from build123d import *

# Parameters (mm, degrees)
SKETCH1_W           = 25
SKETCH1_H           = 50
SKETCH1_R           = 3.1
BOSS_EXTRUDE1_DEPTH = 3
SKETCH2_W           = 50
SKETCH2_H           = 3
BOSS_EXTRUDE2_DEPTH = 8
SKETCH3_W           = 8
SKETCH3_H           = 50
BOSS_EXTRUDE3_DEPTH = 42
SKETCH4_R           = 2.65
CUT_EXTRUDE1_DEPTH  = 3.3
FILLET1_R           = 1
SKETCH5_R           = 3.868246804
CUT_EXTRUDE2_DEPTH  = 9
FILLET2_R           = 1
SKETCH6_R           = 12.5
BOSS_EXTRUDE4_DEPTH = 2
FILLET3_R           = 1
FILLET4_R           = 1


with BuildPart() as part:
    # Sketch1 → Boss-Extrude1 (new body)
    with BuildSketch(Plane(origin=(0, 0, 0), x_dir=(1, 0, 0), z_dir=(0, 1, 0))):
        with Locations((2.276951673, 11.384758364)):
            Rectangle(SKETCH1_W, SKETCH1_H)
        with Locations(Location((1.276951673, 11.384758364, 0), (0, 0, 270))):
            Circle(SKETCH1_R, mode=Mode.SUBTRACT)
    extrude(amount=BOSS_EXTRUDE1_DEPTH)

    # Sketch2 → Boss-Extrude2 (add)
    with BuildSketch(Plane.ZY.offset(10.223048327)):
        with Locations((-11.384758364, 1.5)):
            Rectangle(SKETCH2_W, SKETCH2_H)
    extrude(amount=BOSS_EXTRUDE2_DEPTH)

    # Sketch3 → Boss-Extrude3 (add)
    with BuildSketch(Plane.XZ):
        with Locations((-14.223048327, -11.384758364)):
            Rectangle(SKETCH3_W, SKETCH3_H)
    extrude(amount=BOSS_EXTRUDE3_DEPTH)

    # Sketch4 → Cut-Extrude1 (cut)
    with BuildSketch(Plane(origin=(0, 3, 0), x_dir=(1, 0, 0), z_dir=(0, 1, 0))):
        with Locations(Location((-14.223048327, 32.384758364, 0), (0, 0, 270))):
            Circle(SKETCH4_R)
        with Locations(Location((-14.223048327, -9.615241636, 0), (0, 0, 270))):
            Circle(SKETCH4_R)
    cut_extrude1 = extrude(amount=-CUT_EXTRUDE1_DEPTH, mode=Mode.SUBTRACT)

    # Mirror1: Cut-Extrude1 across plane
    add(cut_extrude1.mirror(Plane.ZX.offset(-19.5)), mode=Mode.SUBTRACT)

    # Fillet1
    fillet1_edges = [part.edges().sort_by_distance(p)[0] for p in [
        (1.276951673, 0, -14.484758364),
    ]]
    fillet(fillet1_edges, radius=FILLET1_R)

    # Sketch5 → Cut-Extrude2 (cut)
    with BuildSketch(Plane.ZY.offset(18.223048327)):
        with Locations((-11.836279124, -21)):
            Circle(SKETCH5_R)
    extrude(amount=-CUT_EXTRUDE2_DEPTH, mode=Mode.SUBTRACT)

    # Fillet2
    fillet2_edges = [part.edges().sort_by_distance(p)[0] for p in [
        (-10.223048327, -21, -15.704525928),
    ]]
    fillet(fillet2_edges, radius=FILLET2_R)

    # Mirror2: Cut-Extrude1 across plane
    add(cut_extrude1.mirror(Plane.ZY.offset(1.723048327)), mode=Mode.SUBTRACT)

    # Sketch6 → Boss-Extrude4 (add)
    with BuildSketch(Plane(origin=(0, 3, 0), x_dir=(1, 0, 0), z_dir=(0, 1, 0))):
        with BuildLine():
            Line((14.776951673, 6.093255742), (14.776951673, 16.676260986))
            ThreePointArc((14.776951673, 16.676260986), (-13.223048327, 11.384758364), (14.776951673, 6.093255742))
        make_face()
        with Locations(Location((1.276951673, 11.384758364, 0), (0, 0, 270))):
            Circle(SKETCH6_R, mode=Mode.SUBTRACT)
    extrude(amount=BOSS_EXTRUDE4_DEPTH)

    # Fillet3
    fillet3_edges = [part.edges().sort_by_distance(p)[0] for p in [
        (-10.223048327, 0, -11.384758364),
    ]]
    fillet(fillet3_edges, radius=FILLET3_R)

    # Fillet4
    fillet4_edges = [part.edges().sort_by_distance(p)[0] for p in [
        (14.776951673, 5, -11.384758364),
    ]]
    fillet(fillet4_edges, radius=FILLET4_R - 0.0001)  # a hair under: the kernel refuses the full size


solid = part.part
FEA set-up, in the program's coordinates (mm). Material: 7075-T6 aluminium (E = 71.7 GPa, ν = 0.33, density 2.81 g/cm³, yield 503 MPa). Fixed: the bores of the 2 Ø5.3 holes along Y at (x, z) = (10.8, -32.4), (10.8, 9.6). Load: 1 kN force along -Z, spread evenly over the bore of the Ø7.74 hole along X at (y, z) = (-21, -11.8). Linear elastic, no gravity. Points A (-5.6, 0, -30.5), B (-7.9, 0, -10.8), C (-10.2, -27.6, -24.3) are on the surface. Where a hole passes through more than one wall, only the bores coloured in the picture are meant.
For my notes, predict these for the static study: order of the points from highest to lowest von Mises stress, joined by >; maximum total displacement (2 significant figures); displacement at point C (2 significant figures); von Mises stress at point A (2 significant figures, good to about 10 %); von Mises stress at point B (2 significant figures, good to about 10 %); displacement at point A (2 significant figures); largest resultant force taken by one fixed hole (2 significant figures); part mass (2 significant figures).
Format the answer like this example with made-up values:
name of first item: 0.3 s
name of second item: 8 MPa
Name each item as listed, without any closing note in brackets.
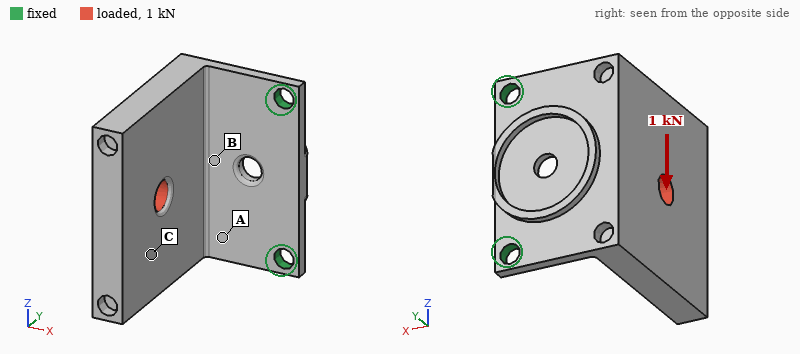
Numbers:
order of the points from highest to lowest von Mises stress, joined by >: A > B > C
maximum total displacement: 0.43 mm
displacement at point C: 0.28 mm
von Mises stress at point A: 110 MPa
von Mises stress at point B: 61 MPa
displacement at point A: 0.12 mm
largest resultant force taken by one fixed hole: 940 N
part mass: 60 g
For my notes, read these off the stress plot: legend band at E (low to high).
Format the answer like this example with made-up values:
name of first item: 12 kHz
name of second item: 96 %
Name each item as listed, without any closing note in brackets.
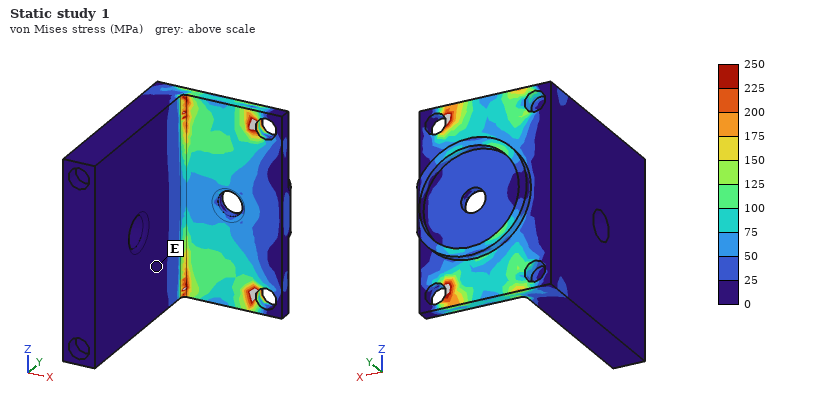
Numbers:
legend band at E: 0 to 25 MPa
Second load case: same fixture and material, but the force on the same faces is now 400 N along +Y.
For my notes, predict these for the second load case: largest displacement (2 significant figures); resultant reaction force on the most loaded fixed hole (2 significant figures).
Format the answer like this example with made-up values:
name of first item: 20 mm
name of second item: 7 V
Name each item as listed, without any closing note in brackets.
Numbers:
largest displacement: 0.74 mm
resultant reaction force on the most loaded fixed hole: 210 N
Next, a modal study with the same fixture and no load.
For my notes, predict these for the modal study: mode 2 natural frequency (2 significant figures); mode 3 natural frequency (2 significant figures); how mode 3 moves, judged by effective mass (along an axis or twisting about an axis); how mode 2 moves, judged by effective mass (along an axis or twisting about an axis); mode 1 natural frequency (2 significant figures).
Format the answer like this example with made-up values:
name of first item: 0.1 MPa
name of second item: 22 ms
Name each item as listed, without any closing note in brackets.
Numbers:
mode 2 natural frequency: 1300 Hz
mode 3 natural frequency: 2200 Hz
how mode 3 moves, judged by effective mass: along Y
how mode 2 moves, judged by effective mass: along Z
mode 1 natural frequency: 490 Hz
